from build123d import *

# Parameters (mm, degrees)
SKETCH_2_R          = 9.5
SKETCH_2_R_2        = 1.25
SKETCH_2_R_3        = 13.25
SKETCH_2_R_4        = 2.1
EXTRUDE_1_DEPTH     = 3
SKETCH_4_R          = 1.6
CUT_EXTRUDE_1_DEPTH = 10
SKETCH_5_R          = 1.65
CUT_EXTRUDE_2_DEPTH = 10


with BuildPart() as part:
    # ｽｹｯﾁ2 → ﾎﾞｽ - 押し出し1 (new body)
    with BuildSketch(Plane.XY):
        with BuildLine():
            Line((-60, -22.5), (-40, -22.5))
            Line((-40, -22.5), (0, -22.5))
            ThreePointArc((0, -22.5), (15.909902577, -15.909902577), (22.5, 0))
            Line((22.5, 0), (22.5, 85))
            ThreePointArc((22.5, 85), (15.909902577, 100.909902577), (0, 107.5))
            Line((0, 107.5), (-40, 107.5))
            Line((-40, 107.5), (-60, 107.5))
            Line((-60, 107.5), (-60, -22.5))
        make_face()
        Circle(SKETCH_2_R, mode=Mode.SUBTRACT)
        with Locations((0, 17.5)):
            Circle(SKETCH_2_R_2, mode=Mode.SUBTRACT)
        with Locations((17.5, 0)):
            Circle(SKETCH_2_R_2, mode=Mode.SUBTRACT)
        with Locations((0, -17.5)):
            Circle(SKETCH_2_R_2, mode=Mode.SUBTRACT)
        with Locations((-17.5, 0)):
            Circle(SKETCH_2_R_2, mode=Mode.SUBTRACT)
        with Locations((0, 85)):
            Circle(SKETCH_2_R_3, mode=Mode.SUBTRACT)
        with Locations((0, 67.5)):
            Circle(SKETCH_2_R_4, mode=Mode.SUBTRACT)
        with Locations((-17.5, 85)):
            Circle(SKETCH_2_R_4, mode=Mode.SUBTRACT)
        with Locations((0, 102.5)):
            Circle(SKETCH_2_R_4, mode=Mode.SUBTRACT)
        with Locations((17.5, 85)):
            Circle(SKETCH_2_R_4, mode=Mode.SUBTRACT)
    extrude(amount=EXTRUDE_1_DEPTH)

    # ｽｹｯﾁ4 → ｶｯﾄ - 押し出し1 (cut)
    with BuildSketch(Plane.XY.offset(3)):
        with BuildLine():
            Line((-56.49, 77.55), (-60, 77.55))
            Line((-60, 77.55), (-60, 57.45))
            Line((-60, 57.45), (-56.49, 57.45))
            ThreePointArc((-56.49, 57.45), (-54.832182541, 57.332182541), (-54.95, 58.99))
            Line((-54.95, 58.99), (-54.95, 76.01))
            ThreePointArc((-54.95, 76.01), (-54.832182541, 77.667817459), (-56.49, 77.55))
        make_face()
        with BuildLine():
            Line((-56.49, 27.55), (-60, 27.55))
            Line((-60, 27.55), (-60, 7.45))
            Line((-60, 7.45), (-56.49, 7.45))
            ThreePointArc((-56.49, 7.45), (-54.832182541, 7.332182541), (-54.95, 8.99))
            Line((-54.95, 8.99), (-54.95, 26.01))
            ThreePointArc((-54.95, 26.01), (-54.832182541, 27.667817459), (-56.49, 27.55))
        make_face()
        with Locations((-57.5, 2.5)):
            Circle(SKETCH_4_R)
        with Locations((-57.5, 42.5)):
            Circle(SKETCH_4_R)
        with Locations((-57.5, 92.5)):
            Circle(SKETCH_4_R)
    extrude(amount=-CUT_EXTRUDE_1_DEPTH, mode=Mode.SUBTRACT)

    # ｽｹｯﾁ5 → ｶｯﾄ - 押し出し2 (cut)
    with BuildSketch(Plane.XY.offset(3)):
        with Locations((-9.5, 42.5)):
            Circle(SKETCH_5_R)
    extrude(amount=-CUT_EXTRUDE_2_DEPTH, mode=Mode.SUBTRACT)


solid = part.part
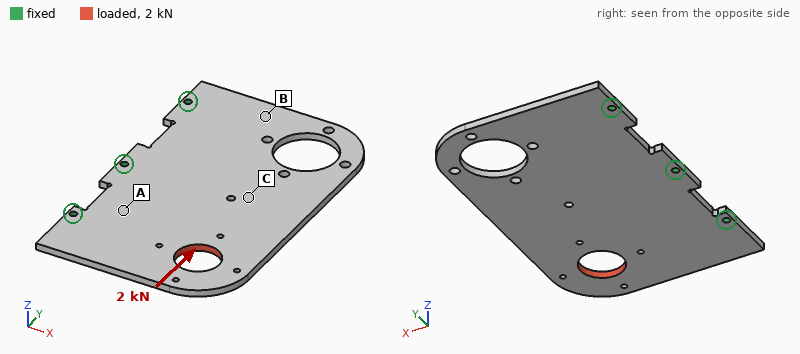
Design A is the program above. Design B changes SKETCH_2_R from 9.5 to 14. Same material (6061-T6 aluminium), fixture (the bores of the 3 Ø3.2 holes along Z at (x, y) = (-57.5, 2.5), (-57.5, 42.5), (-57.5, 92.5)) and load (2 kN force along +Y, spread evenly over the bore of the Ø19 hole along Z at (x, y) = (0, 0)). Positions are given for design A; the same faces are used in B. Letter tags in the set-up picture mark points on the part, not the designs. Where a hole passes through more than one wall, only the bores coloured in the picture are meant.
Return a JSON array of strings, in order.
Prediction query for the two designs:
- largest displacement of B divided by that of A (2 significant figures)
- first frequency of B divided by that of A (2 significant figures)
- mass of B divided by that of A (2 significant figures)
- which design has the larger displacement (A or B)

["1.2", "1.0", "0.96", "B"]
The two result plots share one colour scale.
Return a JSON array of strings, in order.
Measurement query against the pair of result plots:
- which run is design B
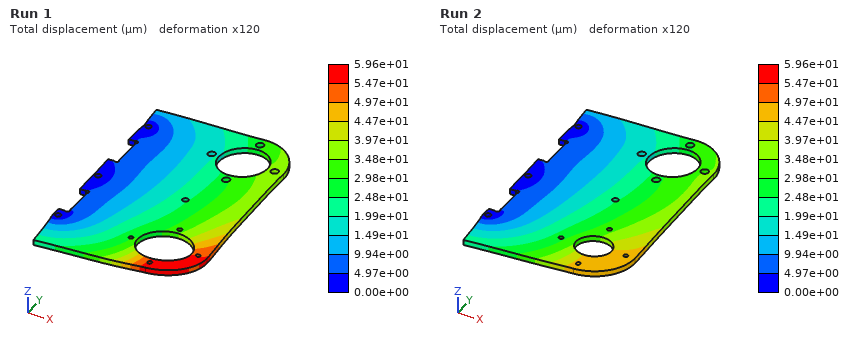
["Run 1"]
